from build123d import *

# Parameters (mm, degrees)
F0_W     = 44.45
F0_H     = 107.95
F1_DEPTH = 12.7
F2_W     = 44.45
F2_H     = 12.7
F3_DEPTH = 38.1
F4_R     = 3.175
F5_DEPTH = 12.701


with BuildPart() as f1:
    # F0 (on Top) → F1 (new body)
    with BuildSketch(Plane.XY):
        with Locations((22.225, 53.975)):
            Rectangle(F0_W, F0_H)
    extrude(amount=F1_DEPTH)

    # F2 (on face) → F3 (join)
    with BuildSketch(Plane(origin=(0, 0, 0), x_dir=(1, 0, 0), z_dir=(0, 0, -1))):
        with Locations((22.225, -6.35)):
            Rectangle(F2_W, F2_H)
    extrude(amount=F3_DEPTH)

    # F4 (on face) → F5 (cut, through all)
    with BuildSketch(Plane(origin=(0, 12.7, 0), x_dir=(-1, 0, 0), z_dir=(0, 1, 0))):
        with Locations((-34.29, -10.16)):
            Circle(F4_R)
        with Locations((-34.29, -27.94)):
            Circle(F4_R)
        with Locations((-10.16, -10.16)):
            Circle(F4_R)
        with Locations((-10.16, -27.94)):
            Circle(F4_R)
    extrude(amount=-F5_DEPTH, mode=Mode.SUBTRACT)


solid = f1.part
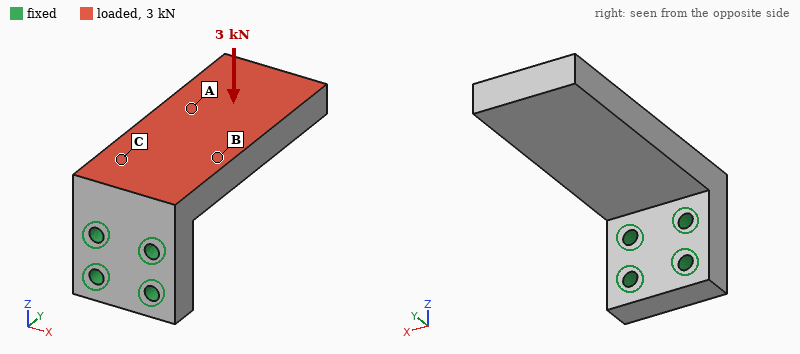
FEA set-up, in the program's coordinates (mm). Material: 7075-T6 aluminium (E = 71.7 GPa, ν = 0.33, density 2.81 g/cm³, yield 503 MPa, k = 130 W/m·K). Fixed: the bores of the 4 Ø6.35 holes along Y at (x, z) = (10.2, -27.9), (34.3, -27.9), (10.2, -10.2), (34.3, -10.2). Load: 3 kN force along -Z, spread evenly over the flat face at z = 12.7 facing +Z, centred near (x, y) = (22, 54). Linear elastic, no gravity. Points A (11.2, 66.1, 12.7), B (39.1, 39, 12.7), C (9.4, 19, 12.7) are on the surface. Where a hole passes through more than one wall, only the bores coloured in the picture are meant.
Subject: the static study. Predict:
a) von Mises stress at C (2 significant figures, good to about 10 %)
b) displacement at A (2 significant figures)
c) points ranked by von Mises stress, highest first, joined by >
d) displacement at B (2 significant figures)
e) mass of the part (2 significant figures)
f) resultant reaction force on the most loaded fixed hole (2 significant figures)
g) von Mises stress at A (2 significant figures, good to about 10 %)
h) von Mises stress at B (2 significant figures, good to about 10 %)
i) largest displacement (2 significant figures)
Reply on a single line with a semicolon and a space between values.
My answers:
90 MPa; 0.50 mm; C > B > A; 0.23 mm; 230 g; 1.7 kN; 21 MPa; 56 MPa; 0.99 mm
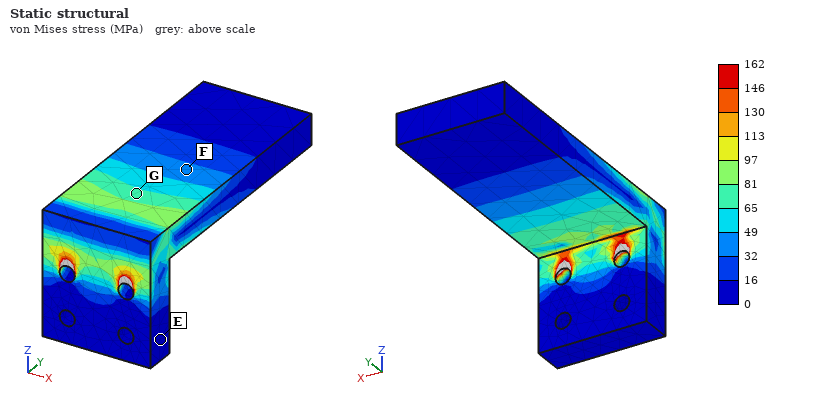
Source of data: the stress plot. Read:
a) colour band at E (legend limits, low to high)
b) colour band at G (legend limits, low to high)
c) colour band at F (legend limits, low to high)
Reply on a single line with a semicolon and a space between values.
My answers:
0 to 16 MPa; 65 to 81 MPa; 32 to 49 MPa
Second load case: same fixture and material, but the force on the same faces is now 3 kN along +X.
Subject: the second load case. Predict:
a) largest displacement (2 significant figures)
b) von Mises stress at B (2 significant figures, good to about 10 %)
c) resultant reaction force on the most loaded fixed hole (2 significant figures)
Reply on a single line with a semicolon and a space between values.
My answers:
0.19 mm; 15 MPa; 5.0 kN
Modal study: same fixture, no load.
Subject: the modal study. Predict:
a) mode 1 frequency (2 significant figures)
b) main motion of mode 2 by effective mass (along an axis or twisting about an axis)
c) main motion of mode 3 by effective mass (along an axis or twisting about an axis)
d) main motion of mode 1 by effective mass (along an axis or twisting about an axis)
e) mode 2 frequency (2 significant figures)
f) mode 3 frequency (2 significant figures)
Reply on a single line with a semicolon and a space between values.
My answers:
830 Hz; along X; twisting about Y; along Z; 1900 Hz; 4100 Hz
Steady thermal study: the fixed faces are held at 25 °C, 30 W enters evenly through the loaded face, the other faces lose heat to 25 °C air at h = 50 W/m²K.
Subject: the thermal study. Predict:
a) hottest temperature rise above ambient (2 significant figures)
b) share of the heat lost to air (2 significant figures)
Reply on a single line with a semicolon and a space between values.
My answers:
19 K; 19 %
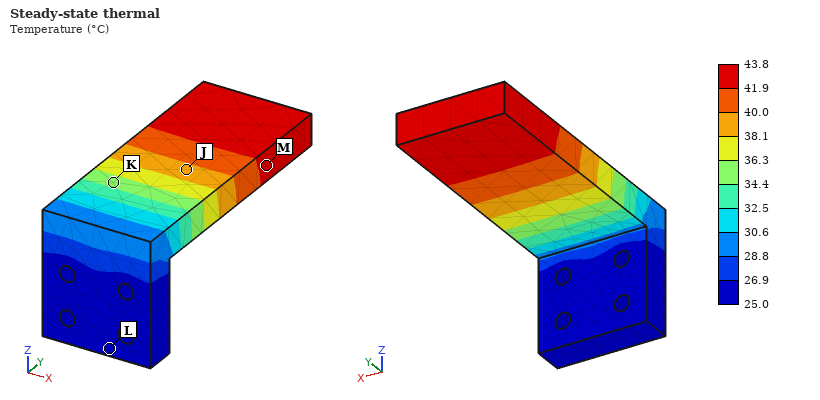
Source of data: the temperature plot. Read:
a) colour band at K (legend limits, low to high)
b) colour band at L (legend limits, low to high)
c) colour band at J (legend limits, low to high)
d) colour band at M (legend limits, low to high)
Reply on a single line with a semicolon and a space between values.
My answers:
34.4 to 36.3 °C; 25.0 to 26.9 °C; 38.1 to 40.0 °C; 41.9 to 43.8 °C
